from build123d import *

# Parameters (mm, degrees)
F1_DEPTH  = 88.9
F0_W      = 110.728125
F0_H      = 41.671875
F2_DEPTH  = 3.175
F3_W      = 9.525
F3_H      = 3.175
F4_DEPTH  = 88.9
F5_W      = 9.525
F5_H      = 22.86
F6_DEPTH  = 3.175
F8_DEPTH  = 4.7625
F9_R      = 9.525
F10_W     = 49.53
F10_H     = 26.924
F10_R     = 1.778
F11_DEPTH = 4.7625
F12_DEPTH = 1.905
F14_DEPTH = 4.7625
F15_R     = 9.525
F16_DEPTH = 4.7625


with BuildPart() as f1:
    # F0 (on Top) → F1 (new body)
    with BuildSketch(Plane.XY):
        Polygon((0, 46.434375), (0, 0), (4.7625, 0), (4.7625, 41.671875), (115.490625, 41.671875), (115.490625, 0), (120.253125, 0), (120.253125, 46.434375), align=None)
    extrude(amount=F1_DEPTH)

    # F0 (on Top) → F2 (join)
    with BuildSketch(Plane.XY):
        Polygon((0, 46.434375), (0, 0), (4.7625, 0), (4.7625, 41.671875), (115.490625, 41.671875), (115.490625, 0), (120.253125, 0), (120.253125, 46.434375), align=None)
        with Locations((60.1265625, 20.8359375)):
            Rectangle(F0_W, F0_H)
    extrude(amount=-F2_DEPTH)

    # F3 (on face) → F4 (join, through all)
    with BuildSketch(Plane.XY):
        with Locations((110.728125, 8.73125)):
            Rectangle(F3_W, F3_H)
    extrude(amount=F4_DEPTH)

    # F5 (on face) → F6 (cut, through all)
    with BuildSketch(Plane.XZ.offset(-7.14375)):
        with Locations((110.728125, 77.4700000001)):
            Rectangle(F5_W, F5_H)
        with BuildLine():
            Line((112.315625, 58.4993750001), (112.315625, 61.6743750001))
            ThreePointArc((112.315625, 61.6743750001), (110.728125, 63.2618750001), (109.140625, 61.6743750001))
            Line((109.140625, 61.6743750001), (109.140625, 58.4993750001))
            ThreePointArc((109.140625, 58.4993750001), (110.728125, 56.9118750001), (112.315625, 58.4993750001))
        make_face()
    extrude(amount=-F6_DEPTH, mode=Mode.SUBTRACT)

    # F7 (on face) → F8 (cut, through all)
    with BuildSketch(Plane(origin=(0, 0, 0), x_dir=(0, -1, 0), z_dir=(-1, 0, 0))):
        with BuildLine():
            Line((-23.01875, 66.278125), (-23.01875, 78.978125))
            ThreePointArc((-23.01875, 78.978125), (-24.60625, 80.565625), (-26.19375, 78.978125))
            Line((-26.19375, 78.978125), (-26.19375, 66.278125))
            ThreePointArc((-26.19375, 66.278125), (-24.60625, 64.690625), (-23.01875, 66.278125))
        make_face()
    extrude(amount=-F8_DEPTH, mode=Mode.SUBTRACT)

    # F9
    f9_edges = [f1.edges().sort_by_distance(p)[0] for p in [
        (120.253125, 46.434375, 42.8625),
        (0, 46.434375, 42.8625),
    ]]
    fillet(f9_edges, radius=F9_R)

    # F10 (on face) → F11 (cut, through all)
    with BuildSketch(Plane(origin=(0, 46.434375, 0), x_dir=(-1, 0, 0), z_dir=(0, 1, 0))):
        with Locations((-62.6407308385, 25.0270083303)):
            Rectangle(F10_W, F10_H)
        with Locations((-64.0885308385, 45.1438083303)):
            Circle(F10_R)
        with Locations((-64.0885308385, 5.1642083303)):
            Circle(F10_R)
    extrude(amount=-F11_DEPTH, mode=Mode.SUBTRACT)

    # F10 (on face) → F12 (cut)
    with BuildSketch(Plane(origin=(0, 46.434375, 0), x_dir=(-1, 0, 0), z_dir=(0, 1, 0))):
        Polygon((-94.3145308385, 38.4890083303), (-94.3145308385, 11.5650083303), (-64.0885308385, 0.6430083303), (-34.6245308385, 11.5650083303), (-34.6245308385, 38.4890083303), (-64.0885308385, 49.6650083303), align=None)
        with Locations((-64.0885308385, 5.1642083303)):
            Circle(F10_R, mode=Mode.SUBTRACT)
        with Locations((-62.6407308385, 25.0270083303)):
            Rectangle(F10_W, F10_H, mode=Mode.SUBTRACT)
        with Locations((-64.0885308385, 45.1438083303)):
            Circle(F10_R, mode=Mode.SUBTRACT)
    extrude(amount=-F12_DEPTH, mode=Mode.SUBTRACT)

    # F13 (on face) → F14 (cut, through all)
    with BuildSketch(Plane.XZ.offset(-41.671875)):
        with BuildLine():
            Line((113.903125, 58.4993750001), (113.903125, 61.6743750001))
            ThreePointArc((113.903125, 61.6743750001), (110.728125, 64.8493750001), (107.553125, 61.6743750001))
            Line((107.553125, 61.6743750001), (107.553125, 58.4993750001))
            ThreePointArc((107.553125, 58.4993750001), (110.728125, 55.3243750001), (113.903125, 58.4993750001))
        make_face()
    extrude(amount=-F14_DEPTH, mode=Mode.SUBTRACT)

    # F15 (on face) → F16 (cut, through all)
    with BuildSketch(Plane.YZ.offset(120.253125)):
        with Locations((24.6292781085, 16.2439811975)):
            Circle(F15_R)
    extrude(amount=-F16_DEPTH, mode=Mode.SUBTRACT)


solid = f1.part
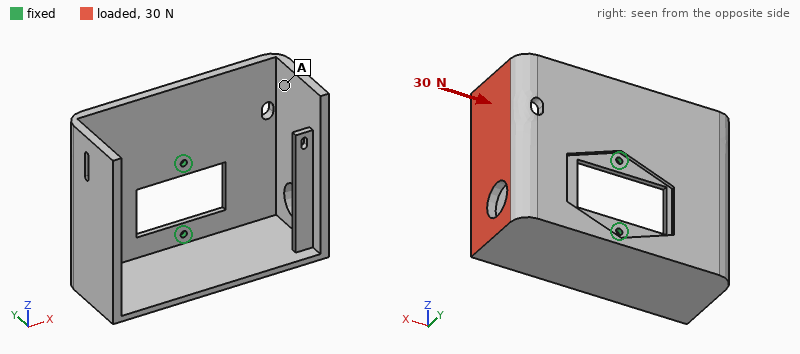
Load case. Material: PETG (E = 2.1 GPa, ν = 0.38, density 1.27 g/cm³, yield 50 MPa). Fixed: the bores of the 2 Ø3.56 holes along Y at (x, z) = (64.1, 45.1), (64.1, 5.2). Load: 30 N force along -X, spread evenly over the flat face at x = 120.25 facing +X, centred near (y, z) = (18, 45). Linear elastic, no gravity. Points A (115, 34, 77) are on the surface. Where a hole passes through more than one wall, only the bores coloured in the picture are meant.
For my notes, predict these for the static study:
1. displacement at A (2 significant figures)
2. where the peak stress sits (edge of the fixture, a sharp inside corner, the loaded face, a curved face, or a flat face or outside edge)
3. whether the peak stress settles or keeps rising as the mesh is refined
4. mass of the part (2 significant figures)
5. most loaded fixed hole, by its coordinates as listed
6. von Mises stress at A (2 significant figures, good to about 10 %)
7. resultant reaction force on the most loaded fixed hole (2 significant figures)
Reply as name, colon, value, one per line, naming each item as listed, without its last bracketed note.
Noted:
displacement at A: 0.81 mm
where the peak stress sits: edge of the fixture
whether the peak stress settles or keeps rising as the mesh is refined: keeps rising
mass of the part: 120 g
most loaded fixed hole, by its coordinates as listed: (64.1, 45.1)
von Mises stress at A: 0.86 MPa
resultant reaction force on the most loaded fixed hole: 30 N
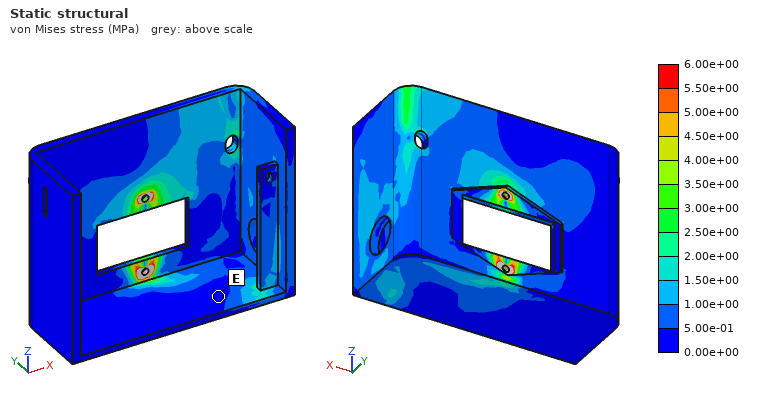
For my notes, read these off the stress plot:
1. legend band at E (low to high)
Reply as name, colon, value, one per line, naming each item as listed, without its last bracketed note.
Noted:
legend band at E: 0.00e+00 to 5.00e-01 MPa
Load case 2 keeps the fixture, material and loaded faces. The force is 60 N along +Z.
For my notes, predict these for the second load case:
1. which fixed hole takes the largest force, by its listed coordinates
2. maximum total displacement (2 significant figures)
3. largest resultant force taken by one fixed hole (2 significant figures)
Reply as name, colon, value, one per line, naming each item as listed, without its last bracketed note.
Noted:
which fixed hole takes the largest force, by its listed coordinates: (64.1, 45.1)
maximum total displacement: 1.5 mm
largest resultant force taken by one fixed hole: 93 N
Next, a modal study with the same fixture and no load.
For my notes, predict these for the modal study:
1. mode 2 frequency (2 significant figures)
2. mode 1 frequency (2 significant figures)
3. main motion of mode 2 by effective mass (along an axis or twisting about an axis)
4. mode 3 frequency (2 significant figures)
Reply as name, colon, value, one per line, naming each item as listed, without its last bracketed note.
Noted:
mode 2 frequency: 140 Hz
mode 1 frequency: 71 Hz
main motion of mode 2 by effective mass: along Y
mode 3 frequency: 170 Hz
